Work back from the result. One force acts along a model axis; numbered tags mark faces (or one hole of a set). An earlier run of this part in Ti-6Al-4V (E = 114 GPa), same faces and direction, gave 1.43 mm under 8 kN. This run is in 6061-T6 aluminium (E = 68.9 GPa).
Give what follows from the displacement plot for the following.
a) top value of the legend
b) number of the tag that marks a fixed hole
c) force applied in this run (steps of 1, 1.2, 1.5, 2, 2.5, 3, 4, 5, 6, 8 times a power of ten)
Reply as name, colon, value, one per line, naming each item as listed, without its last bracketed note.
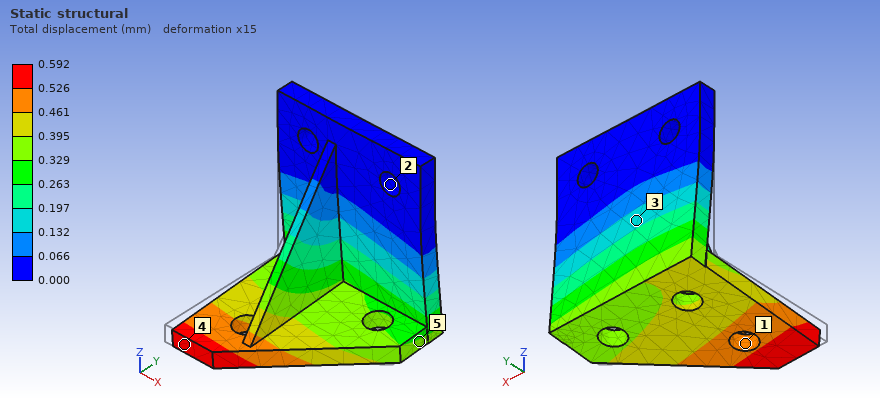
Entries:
top value of the legend: 0.592 mm
number of the tag that marks a fixed hole: 2
force applied in this run: 2 kN
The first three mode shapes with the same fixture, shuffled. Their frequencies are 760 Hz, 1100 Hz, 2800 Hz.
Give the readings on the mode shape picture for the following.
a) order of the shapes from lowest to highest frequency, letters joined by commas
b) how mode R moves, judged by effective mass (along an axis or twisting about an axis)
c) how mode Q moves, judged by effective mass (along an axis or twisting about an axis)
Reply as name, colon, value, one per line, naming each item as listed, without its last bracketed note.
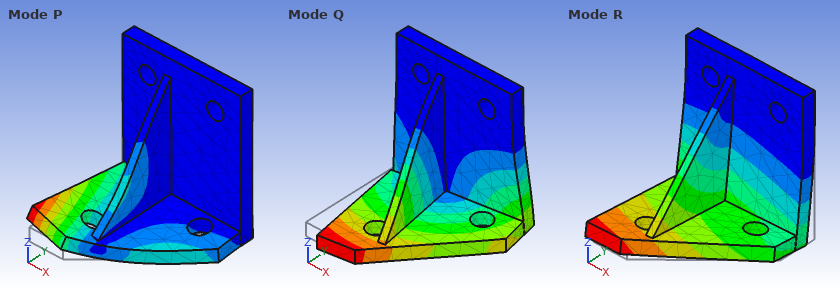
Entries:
order of the shapes from lowest to highest frequency, letters joined by commas: R, Q, P
how mode R moves, judged by effective mass: along Y
how mode Q moves, judged by effective mass: along X
